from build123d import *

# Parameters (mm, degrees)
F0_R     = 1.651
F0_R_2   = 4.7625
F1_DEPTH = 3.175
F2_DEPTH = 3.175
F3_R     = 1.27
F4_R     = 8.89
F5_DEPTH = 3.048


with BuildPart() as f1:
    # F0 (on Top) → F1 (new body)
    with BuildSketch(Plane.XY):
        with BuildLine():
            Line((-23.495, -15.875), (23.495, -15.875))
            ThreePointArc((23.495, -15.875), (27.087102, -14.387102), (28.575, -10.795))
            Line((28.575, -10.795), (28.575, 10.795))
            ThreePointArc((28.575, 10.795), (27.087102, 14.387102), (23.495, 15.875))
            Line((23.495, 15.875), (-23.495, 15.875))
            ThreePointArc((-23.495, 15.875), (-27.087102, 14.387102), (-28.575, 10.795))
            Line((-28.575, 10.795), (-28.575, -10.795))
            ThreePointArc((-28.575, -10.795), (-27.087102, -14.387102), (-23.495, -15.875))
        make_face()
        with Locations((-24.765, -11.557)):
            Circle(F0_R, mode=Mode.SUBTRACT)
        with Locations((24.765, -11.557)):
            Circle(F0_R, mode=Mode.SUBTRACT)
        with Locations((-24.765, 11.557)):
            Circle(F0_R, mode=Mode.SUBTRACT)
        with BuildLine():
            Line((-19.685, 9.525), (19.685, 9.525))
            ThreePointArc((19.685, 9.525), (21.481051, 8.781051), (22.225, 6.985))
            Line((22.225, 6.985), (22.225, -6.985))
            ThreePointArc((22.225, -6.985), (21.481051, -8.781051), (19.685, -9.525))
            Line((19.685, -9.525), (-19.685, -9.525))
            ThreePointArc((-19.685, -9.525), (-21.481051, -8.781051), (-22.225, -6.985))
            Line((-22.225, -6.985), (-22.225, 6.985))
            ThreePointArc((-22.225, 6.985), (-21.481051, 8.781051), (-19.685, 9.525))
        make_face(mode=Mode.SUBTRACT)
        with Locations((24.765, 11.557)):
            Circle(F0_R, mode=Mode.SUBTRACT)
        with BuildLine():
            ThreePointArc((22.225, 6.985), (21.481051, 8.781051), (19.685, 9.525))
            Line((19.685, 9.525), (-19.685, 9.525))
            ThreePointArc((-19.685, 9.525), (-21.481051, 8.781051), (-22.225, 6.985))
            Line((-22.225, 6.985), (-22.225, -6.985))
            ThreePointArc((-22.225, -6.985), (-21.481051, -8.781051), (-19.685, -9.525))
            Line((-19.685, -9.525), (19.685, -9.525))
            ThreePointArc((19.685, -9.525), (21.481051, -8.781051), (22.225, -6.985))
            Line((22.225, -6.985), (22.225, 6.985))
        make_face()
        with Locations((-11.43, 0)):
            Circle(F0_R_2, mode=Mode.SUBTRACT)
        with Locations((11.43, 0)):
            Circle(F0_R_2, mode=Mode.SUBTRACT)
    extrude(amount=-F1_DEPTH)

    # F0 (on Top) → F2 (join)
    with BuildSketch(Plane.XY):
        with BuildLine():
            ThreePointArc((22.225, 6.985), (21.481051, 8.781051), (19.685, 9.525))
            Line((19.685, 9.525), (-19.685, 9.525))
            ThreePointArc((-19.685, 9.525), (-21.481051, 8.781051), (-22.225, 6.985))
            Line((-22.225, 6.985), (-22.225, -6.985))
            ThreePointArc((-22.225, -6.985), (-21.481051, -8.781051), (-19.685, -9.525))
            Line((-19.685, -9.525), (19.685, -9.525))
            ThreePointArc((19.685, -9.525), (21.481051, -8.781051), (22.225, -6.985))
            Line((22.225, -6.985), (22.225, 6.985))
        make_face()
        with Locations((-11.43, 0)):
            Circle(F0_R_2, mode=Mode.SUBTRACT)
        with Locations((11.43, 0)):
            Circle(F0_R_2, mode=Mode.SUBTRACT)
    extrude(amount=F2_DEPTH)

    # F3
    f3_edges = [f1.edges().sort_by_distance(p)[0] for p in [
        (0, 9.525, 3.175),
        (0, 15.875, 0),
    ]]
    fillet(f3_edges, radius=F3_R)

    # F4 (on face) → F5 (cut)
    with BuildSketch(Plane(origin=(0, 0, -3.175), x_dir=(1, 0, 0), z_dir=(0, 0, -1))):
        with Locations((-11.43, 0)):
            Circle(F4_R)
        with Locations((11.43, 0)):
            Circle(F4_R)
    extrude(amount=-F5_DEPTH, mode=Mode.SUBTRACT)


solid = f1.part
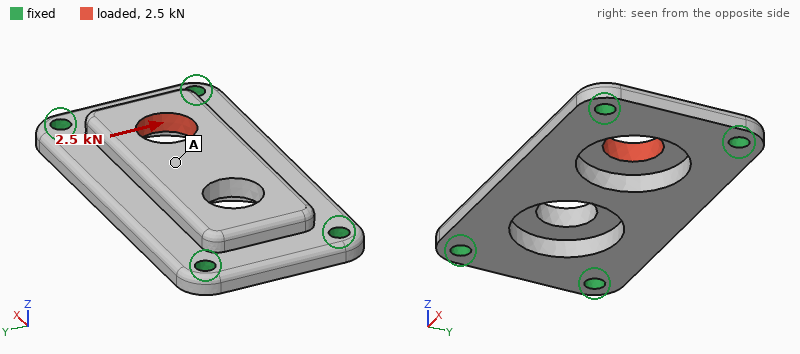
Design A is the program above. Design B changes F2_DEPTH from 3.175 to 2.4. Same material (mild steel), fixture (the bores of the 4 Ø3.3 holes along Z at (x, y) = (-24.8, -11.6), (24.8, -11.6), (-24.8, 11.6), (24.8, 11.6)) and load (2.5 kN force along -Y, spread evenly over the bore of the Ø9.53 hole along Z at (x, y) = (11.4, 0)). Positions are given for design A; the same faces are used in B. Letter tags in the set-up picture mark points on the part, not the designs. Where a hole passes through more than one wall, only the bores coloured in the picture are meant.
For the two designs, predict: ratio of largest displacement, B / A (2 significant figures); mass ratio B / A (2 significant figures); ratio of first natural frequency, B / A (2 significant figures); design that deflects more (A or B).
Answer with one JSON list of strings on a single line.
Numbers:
["1.1", "0.91", "0.94", "B"]
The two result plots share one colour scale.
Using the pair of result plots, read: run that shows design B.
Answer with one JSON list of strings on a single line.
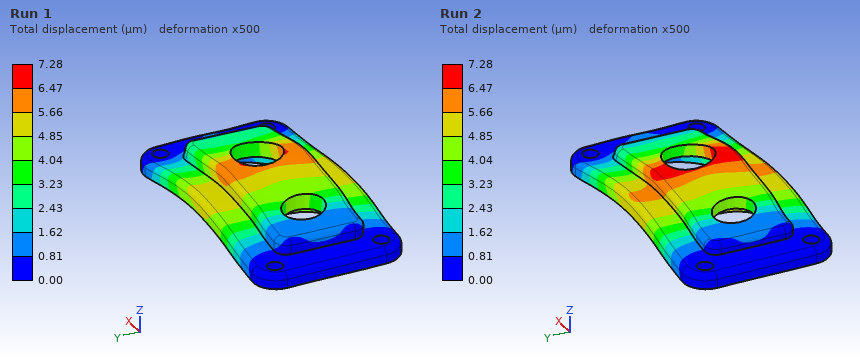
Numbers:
["Run 2"]
